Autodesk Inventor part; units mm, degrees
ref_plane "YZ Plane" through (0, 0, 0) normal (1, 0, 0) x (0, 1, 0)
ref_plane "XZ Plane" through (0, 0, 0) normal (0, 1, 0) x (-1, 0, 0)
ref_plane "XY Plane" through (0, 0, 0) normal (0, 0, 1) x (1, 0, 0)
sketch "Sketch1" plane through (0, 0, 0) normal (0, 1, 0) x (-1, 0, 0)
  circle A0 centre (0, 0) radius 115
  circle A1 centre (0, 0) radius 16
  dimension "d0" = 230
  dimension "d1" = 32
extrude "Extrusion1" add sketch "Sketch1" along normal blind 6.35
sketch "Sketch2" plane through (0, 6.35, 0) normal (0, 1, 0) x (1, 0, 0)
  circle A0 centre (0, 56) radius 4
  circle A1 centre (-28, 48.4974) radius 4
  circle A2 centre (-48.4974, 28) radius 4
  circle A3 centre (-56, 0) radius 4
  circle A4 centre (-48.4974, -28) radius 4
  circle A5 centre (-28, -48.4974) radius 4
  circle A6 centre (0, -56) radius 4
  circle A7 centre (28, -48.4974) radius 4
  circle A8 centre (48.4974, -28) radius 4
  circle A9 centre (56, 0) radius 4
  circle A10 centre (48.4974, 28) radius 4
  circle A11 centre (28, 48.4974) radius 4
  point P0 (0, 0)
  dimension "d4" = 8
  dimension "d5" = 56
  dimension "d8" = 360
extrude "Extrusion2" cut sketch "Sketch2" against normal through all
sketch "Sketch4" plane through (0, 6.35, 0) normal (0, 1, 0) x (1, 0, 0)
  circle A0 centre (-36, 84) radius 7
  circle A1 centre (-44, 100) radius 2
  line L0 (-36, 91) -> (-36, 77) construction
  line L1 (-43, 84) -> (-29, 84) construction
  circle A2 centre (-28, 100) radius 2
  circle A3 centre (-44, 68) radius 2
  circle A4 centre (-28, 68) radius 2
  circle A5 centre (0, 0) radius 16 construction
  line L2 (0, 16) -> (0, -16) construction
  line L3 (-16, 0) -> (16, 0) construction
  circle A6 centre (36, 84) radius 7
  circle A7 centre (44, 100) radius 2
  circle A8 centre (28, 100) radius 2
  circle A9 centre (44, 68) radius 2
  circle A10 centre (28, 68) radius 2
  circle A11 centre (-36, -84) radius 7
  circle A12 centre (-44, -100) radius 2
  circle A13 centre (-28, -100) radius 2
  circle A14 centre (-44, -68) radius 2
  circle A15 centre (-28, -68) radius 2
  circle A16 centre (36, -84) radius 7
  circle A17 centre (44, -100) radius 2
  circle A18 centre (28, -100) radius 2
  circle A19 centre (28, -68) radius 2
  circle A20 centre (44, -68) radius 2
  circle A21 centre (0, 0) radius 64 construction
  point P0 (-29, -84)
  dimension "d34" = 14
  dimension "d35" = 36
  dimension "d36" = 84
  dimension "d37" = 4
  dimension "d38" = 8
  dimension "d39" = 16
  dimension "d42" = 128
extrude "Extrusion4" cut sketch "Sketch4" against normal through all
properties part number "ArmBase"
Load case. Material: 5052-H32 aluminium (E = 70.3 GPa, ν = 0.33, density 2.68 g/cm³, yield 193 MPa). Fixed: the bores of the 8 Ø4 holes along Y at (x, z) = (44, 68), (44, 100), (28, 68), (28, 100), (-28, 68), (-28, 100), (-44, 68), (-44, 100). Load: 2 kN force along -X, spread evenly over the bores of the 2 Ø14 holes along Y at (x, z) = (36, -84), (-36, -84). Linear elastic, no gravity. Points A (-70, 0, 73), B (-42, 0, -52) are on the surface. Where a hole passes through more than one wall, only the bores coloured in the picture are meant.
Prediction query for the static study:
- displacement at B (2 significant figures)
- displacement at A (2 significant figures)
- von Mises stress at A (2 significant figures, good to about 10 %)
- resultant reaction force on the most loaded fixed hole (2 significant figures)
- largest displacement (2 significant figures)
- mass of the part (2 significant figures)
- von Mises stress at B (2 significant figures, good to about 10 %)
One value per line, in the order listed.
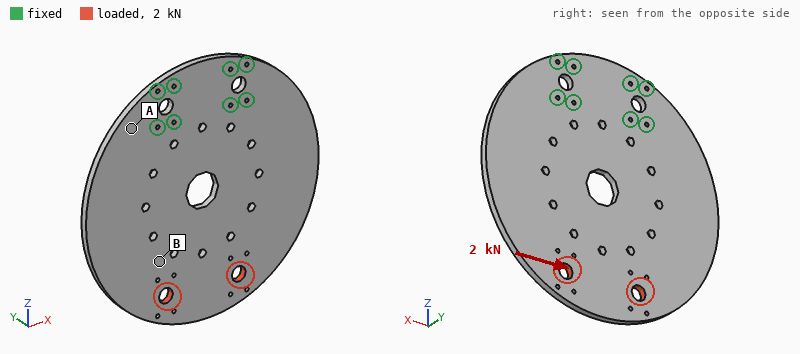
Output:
35 µm
8.0 µm
7.1 MPa
1.9 kN
49 µm
670 g
3.3 MPa
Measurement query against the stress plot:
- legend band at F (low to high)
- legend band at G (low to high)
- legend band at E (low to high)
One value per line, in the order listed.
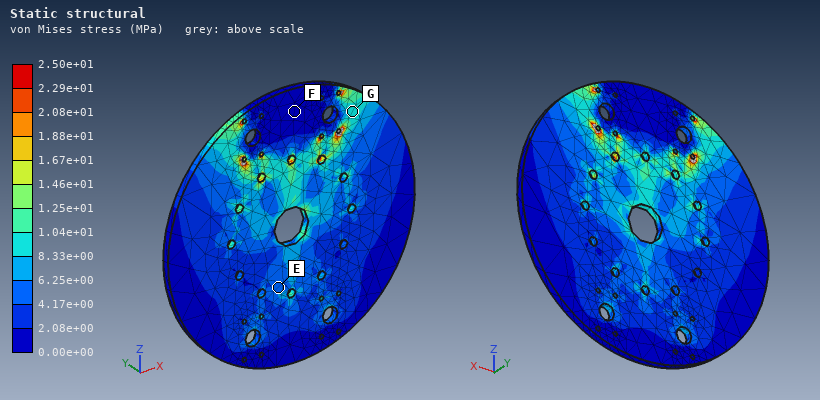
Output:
0.00e+00 to 2.08e+00 MPa
8.33e+00 to 1.04e+01 MPa
4.17e+00 to 6.25e+00 MPa
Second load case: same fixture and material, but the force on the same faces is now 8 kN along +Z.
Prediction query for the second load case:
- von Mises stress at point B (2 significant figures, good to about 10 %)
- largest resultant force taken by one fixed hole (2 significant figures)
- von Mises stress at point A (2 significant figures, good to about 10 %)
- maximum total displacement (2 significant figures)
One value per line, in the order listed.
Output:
10 MPa
1.9 kN
5.4 MPa
29 µm
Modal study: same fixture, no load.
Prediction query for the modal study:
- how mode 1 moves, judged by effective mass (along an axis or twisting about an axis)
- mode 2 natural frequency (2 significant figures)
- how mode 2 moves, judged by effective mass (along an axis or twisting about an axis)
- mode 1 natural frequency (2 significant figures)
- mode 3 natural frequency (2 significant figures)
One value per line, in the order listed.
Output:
along Y
360 Hz
twisting about Z
170 Hz
730 Hz
